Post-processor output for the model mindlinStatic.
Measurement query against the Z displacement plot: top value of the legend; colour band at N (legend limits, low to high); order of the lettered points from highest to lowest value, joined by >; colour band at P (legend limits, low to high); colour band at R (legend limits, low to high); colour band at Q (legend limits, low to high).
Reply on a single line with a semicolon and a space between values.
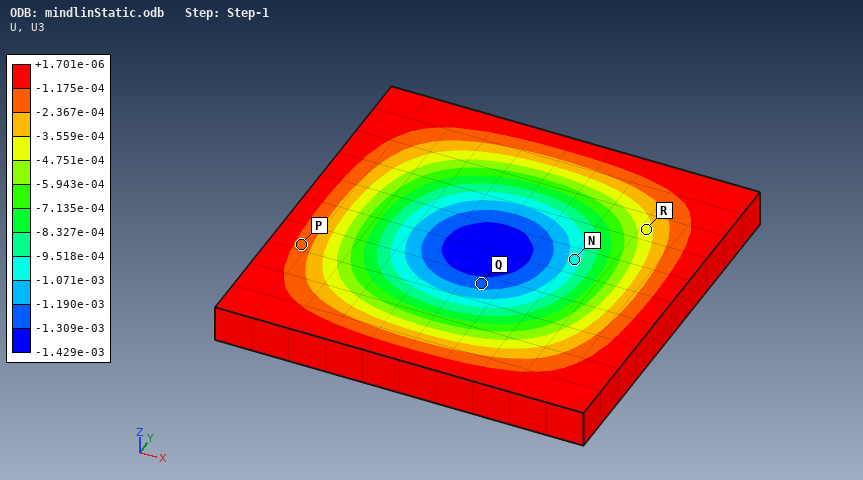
+1.701e-06; -1.071e-03 to -9.518e-04; P > R > N > Q; -2.367e-04 to -1.175e-04; -4.751e-04 to -3.559e-04; -1.309e-03 to -1.190e-03
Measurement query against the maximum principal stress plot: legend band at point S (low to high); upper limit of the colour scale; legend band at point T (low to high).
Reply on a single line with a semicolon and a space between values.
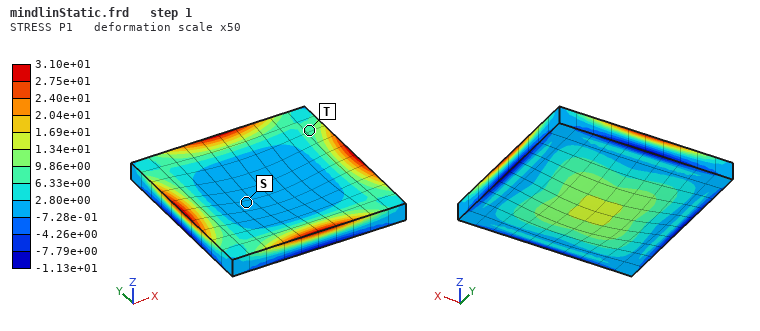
-7.28e-01 to 2.80e+00; 3.10e+01; 6.33e+00 to 9.86e+00
